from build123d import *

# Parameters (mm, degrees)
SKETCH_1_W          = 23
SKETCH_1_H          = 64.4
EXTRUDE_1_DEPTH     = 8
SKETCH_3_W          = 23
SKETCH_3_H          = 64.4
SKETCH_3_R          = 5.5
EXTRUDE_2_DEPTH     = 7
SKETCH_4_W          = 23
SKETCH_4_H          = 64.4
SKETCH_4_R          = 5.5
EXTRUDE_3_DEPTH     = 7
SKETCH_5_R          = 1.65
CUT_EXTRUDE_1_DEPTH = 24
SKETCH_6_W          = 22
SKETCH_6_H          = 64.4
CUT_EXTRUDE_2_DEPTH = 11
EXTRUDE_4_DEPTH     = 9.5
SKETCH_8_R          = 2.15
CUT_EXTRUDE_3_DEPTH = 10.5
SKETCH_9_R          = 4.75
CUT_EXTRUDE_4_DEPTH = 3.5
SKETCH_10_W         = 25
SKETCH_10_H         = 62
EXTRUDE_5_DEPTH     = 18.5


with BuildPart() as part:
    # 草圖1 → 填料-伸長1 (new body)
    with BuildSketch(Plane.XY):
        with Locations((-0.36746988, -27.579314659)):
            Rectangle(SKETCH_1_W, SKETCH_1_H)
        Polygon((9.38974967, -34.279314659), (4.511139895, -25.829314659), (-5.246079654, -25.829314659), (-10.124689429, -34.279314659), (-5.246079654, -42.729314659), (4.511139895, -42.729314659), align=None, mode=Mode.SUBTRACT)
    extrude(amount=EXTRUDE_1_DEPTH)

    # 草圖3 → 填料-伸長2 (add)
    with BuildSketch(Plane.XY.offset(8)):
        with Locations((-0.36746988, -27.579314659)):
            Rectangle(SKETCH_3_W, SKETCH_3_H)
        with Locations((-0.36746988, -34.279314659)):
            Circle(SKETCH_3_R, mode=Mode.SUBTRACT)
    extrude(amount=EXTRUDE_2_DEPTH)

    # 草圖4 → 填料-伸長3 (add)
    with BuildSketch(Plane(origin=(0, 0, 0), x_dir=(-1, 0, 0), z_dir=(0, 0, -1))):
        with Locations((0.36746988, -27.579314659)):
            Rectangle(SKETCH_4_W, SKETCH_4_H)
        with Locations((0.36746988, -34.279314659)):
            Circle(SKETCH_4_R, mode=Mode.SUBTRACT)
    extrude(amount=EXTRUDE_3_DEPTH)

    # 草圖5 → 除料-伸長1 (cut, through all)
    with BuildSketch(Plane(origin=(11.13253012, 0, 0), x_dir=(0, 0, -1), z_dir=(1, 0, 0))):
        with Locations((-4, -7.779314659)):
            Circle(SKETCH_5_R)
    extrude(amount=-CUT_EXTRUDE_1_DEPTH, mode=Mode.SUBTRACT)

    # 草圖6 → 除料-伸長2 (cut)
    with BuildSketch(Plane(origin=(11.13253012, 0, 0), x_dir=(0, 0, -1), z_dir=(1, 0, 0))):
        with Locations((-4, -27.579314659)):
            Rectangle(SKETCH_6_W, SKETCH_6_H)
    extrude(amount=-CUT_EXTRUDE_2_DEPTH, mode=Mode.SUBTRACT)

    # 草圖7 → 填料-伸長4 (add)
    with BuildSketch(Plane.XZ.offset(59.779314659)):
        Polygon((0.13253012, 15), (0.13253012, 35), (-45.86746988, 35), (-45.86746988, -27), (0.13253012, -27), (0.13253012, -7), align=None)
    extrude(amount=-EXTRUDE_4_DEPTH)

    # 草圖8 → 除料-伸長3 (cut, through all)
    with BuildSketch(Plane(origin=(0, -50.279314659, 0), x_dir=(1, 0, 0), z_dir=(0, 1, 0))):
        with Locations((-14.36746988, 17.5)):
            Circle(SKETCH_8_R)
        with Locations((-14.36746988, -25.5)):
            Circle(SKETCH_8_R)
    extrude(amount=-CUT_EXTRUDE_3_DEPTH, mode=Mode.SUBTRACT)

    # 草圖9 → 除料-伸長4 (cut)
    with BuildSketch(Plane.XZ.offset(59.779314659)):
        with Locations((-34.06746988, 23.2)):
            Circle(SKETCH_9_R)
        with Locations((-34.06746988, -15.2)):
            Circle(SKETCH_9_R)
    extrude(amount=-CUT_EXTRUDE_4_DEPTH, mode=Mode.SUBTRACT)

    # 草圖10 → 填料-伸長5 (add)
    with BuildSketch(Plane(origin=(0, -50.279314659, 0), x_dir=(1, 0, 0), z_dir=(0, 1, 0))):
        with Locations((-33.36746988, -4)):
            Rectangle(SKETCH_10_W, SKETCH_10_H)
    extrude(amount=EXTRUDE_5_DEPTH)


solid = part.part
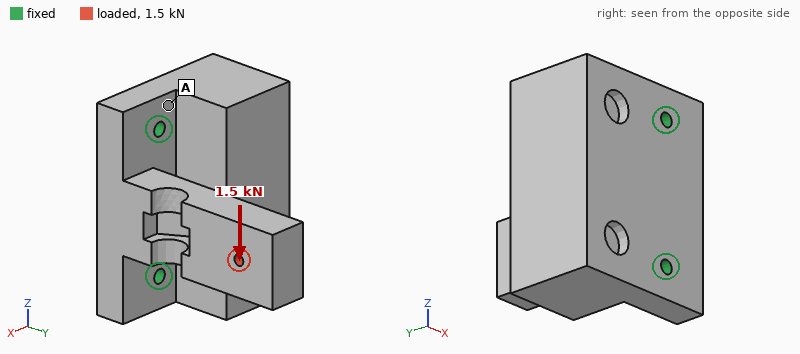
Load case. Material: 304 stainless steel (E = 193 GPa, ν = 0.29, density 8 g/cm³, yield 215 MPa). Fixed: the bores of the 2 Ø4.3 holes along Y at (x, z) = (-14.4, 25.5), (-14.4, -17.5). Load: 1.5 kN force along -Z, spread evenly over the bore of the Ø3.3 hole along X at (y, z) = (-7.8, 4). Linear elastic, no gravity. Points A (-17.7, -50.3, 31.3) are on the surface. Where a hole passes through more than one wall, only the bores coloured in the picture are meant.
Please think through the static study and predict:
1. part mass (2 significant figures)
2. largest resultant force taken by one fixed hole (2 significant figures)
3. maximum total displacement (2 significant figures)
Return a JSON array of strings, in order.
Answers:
["540 g", "2.1 kN", "80 µm"]
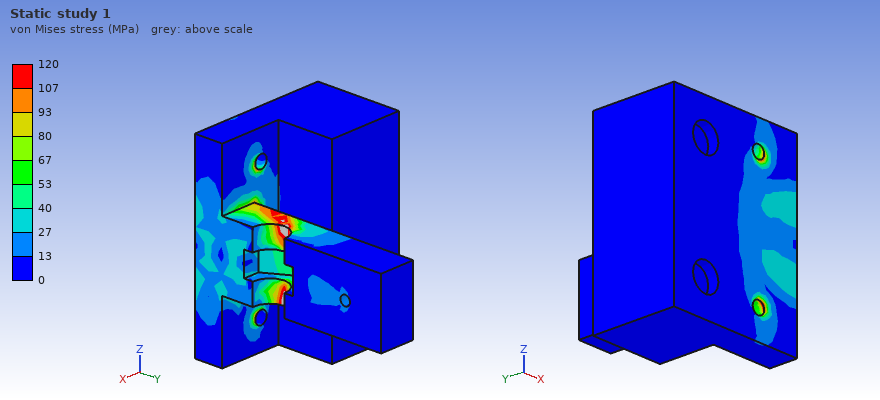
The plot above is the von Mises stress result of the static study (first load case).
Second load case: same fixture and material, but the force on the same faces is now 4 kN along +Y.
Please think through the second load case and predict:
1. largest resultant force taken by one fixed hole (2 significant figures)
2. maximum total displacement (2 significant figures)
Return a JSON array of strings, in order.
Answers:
["2.0 kN", "0.12 mm"]
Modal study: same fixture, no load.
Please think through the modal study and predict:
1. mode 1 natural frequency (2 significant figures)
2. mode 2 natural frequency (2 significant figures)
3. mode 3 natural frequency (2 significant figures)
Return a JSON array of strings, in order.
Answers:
["1400 Hz", "3100 Hz", "3300 Hz"]
